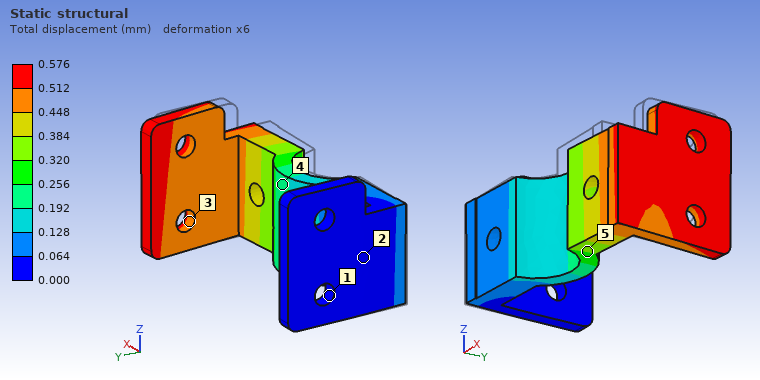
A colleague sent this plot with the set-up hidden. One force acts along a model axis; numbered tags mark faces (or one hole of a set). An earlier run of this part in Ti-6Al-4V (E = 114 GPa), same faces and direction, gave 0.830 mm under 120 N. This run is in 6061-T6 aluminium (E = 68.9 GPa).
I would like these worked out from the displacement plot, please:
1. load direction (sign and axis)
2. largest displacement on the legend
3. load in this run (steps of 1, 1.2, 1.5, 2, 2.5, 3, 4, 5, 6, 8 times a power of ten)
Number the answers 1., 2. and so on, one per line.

1. +Y
2. 0.576 mm
3. 50 N
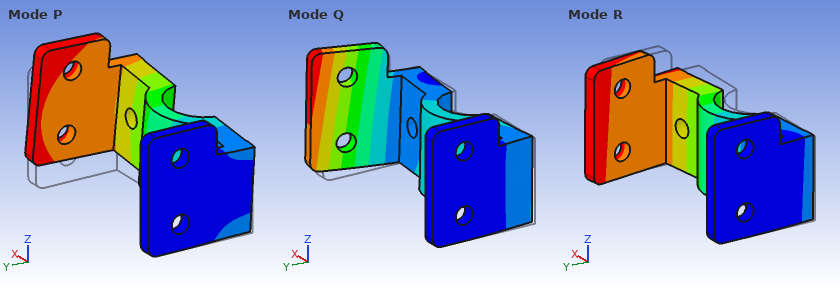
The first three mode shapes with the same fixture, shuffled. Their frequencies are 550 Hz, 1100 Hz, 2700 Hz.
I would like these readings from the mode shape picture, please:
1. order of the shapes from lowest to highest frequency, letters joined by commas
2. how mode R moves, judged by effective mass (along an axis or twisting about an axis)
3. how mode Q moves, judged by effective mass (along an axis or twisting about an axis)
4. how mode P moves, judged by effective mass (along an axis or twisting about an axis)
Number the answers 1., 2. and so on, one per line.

1. R, P, Q
2. along Y
3. along X
4. along Z
